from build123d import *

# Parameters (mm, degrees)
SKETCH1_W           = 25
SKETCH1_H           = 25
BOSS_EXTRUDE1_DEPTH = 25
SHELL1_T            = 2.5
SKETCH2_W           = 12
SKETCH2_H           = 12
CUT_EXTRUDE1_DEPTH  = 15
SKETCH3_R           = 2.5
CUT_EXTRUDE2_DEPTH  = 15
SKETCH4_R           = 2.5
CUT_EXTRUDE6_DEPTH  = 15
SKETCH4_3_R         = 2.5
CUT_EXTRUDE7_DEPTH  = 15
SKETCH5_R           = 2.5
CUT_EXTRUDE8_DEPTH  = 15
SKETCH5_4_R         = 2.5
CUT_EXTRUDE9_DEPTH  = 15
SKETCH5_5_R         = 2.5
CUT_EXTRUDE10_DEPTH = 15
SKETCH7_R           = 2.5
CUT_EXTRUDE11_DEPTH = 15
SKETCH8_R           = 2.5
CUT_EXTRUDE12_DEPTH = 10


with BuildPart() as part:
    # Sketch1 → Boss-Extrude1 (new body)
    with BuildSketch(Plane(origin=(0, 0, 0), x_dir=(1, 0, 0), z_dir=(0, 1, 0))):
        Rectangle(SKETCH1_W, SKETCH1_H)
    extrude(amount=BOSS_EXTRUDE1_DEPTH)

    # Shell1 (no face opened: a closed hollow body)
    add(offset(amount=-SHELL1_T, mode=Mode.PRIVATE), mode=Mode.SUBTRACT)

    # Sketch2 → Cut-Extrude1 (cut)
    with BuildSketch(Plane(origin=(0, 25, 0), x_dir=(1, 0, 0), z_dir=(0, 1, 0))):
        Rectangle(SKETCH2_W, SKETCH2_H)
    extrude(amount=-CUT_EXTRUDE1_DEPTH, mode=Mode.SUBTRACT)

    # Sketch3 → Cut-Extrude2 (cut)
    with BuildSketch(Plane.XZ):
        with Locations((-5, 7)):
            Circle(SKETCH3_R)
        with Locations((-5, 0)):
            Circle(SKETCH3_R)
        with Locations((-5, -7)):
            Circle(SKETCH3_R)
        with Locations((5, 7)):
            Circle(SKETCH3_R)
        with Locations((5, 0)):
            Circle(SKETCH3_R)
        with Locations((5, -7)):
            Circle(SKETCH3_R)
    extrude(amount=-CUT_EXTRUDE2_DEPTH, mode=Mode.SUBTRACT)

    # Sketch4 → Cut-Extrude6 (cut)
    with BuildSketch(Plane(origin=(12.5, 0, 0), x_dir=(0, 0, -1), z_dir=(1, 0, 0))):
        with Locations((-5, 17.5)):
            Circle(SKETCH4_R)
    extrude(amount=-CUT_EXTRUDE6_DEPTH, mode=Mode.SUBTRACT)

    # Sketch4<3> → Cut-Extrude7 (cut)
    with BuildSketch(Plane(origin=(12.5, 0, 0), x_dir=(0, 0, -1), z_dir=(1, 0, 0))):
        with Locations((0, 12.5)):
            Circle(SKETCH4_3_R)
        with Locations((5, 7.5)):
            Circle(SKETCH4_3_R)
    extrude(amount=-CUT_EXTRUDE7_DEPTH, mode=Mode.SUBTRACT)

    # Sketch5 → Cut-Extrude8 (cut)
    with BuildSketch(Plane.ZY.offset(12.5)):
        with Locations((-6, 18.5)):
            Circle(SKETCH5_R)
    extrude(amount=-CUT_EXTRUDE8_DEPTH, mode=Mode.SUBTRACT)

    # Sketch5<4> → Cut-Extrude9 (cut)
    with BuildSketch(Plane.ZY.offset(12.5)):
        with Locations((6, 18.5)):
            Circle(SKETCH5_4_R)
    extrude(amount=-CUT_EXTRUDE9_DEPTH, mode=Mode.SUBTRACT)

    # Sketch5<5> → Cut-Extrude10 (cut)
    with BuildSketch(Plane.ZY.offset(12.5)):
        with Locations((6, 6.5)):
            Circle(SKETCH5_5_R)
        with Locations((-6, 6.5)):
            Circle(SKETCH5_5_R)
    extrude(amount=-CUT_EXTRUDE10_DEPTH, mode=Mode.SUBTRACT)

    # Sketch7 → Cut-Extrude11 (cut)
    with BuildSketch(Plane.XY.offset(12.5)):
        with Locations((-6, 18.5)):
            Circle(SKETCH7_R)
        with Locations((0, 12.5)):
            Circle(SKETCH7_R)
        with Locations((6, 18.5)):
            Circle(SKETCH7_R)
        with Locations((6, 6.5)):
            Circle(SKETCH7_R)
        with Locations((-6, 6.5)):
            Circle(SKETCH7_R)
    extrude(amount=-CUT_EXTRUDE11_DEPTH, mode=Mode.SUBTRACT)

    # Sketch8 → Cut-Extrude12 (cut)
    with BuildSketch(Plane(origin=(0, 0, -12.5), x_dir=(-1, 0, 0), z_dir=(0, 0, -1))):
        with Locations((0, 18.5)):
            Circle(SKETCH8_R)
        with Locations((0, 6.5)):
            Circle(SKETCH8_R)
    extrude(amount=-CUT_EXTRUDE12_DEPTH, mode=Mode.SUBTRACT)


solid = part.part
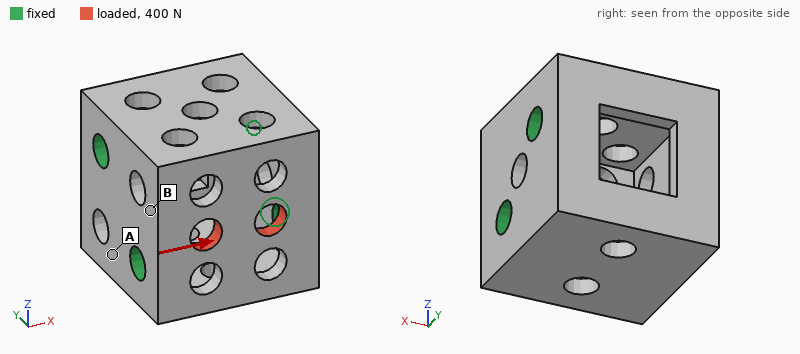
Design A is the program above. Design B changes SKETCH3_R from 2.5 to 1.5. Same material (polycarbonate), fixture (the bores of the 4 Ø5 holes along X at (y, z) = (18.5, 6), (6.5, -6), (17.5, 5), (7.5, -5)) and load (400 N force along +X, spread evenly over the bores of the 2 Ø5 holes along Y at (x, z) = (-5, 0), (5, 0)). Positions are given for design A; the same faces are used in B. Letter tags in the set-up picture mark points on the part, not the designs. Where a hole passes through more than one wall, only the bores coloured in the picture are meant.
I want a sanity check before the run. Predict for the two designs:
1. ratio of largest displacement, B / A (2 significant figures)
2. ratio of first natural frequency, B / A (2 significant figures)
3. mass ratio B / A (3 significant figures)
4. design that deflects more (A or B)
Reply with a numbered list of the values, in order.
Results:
1. 0.81
2. 1.0
3. 1.03
4. A
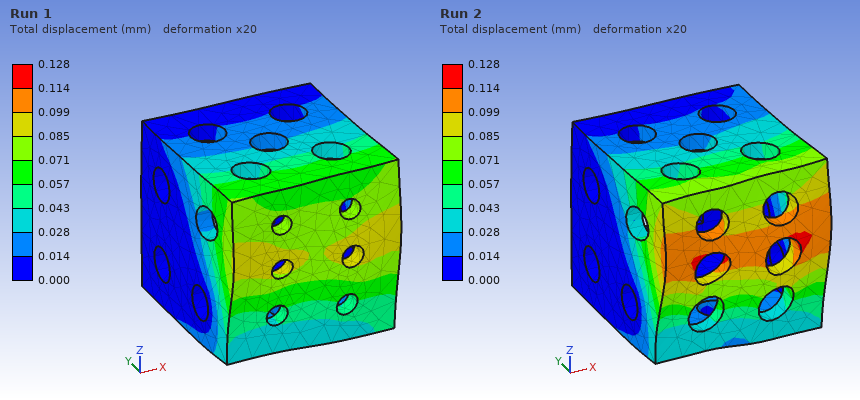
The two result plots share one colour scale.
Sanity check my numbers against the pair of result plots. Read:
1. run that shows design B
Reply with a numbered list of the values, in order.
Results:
1. Run 1
